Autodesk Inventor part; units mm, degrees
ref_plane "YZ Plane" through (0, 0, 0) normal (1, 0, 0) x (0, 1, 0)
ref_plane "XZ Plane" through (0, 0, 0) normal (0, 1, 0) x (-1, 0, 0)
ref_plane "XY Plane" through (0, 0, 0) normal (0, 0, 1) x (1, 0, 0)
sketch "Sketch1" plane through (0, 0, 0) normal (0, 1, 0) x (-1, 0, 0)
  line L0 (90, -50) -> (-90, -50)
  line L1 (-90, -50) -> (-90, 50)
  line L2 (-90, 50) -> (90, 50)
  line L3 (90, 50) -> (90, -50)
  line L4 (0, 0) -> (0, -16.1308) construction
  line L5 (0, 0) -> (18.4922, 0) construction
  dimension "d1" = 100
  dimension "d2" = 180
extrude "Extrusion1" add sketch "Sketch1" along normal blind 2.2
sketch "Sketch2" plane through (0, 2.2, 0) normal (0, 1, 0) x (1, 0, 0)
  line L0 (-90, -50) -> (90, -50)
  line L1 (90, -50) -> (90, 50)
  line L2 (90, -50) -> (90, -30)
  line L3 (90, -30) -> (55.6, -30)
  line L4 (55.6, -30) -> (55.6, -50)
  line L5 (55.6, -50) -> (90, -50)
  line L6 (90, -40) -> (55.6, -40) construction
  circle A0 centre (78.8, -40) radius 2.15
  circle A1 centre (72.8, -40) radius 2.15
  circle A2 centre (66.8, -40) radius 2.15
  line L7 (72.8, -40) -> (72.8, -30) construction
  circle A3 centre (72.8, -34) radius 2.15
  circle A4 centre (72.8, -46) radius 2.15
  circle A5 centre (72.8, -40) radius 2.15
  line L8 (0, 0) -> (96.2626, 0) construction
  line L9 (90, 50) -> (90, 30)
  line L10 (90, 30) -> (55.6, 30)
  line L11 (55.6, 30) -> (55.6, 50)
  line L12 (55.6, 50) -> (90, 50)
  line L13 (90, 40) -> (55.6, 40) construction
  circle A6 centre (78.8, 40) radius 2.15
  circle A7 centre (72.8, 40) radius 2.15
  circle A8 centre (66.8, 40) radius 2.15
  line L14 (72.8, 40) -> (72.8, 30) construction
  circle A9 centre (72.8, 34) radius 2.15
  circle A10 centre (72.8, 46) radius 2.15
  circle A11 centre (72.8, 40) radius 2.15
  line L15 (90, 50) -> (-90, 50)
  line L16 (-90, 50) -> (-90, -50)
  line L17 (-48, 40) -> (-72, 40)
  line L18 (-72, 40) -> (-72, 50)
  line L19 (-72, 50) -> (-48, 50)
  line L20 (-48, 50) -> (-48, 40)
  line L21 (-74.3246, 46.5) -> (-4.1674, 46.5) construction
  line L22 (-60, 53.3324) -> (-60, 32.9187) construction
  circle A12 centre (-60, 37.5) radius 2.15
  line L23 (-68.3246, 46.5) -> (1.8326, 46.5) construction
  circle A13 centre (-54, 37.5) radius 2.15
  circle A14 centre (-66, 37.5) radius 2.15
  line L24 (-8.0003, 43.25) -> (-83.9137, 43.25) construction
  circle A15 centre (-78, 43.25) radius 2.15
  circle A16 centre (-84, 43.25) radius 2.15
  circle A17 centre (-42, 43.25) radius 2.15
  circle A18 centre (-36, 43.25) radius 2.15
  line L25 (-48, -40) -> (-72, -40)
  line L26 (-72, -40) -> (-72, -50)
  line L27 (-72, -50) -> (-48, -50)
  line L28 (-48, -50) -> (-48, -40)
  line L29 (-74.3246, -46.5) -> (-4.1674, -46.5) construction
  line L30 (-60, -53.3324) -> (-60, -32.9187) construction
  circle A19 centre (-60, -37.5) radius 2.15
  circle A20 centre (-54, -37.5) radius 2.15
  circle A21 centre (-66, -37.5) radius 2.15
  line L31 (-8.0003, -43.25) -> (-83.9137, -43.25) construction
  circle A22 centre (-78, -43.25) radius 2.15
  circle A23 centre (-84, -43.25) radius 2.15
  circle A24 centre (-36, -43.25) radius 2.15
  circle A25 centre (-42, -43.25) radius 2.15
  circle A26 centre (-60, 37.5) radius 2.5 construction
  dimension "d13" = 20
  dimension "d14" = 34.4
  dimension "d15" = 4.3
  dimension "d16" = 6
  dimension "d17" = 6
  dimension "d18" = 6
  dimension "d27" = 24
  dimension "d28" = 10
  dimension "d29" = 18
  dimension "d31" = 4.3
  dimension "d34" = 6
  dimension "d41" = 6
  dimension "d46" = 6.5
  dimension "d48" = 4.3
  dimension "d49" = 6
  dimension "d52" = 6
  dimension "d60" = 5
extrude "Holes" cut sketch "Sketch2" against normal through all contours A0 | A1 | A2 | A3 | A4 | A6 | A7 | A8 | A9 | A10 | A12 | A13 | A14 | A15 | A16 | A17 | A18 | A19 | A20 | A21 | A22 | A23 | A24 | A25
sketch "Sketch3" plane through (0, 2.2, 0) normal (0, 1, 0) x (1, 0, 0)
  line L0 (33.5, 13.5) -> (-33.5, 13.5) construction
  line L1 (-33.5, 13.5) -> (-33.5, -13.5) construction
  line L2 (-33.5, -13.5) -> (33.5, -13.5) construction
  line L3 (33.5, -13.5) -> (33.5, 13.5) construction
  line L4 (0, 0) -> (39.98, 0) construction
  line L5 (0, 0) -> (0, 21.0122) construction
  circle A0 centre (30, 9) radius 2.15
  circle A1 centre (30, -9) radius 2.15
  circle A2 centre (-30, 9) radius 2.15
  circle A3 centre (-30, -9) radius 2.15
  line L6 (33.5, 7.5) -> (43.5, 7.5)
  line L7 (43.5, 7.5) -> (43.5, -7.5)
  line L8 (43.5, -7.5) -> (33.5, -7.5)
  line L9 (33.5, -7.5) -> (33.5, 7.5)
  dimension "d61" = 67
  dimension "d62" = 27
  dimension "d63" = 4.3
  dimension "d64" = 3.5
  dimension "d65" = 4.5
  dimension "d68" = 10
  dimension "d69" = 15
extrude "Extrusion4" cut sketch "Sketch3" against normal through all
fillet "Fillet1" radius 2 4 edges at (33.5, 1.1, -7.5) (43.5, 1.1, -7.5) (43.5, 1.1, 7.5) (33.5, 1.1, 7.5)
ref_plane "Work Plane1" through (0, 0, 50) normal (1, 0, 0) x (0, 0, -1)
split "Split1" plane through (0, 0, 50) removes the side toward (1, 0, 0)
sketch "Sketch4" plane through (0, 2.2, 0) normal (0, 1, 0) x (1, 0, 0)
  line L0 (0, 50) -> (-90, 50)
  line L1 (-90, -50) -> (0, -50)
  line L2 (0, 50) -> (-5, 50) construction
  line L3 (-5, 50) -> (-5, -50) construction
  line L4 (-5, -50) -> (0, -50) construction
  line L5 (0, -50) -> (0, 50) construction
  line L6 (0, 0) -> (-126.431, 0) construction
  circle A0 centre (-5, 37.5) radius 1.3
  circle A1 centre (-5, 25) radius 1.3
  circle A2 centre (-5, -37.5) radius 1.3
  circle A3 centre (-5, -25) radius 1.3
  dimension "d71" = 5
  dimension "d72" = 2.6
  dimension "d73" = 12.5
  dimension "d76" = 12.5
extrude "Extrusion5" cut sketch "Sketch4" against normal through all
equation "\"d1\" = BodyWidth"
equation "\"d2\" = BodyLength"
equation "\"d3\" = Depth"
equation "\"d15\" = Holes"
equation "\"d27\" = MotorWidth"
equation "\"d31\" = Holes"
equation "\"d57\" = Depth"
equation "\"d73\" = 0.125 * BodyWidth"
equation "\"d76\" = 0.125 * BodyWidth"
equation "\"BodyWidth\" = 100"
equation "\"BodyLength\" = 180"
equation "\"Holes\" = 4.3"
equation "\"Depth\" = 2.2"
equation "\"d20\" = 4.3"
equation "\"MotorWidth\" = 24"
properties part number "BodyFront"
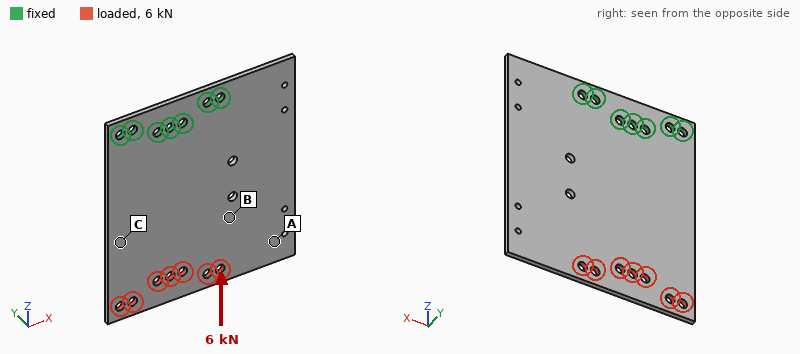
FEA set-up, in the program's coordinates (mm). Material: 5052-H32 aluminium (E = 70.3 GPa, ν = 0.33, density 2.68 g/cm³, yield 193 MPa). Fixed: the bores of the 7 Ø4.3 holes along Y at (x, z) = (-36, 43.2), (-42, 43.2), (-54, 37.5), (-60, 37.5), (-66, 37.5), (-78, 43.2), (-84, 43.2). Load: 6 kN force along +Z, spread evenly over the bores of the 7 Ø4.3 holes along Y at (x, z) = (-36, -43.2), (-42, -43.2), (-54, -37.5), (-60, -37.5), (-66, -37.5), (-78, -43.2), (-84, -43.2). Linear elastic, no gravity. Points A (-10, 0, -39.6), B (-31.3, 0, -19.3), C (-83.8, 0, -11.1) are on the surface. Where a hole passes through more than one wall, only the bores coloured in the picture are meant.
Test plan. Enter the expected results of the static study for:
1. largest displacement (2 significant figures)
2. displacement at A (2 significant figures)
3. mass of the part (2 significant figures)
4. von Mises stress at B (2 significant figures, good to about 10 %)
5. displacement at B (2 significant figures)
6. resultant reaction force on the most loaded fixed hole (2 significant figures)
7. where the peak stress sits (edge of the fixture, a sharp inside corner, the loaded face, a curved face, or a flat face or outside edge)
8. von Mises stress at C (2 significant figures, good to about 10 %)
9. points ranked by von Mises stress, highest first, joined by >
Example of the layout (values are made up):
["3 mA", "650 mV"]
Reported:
["64 µm", "20 µm", "52 g", "22 MPa", "27 µm", "1.1 kN", "the loaded face", "48 MPa", "C > B > A"]
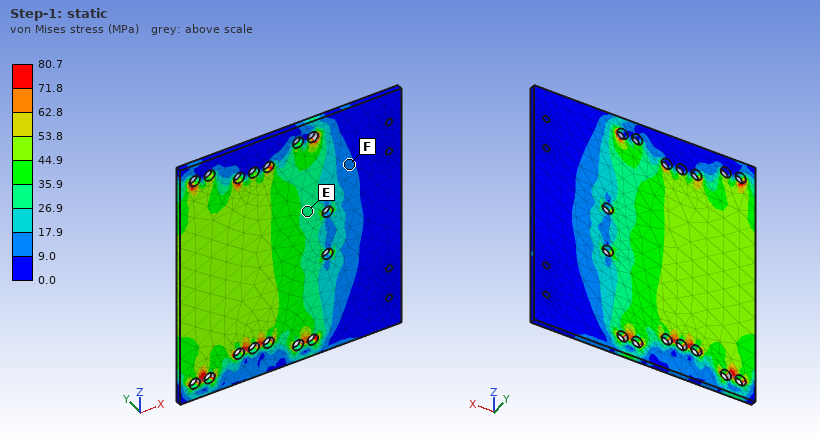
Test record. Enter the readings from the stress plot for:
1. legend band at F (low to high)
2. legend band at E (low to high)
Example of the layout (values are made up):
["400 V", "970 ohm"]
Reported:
["9.0 to 17.9 MPa", "26.9 to 35.9 MPa"]
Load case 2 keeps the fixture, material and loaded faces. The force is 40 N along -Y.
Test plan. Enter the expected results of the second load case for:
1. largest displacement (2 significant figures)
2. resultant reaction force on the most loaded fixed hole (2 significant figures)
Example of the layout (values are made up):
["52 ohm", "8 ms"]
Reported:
["1.5 mm", "49 N"]
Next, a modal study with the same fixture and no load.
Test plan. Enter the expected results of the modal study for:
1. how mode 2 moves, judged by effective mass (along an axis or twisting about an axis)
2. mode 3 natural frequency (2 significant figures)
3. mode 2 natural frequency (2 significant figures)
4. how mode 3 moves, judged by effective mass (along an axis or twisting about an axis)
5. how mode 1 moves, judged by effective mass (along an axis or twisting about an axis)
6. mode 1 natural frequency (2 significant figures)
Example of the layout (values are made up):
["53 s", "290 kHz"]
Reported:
["twisting about Z", "1100 Hz", "490 Hz", "along Y", "along Y", "230 Hz"]
